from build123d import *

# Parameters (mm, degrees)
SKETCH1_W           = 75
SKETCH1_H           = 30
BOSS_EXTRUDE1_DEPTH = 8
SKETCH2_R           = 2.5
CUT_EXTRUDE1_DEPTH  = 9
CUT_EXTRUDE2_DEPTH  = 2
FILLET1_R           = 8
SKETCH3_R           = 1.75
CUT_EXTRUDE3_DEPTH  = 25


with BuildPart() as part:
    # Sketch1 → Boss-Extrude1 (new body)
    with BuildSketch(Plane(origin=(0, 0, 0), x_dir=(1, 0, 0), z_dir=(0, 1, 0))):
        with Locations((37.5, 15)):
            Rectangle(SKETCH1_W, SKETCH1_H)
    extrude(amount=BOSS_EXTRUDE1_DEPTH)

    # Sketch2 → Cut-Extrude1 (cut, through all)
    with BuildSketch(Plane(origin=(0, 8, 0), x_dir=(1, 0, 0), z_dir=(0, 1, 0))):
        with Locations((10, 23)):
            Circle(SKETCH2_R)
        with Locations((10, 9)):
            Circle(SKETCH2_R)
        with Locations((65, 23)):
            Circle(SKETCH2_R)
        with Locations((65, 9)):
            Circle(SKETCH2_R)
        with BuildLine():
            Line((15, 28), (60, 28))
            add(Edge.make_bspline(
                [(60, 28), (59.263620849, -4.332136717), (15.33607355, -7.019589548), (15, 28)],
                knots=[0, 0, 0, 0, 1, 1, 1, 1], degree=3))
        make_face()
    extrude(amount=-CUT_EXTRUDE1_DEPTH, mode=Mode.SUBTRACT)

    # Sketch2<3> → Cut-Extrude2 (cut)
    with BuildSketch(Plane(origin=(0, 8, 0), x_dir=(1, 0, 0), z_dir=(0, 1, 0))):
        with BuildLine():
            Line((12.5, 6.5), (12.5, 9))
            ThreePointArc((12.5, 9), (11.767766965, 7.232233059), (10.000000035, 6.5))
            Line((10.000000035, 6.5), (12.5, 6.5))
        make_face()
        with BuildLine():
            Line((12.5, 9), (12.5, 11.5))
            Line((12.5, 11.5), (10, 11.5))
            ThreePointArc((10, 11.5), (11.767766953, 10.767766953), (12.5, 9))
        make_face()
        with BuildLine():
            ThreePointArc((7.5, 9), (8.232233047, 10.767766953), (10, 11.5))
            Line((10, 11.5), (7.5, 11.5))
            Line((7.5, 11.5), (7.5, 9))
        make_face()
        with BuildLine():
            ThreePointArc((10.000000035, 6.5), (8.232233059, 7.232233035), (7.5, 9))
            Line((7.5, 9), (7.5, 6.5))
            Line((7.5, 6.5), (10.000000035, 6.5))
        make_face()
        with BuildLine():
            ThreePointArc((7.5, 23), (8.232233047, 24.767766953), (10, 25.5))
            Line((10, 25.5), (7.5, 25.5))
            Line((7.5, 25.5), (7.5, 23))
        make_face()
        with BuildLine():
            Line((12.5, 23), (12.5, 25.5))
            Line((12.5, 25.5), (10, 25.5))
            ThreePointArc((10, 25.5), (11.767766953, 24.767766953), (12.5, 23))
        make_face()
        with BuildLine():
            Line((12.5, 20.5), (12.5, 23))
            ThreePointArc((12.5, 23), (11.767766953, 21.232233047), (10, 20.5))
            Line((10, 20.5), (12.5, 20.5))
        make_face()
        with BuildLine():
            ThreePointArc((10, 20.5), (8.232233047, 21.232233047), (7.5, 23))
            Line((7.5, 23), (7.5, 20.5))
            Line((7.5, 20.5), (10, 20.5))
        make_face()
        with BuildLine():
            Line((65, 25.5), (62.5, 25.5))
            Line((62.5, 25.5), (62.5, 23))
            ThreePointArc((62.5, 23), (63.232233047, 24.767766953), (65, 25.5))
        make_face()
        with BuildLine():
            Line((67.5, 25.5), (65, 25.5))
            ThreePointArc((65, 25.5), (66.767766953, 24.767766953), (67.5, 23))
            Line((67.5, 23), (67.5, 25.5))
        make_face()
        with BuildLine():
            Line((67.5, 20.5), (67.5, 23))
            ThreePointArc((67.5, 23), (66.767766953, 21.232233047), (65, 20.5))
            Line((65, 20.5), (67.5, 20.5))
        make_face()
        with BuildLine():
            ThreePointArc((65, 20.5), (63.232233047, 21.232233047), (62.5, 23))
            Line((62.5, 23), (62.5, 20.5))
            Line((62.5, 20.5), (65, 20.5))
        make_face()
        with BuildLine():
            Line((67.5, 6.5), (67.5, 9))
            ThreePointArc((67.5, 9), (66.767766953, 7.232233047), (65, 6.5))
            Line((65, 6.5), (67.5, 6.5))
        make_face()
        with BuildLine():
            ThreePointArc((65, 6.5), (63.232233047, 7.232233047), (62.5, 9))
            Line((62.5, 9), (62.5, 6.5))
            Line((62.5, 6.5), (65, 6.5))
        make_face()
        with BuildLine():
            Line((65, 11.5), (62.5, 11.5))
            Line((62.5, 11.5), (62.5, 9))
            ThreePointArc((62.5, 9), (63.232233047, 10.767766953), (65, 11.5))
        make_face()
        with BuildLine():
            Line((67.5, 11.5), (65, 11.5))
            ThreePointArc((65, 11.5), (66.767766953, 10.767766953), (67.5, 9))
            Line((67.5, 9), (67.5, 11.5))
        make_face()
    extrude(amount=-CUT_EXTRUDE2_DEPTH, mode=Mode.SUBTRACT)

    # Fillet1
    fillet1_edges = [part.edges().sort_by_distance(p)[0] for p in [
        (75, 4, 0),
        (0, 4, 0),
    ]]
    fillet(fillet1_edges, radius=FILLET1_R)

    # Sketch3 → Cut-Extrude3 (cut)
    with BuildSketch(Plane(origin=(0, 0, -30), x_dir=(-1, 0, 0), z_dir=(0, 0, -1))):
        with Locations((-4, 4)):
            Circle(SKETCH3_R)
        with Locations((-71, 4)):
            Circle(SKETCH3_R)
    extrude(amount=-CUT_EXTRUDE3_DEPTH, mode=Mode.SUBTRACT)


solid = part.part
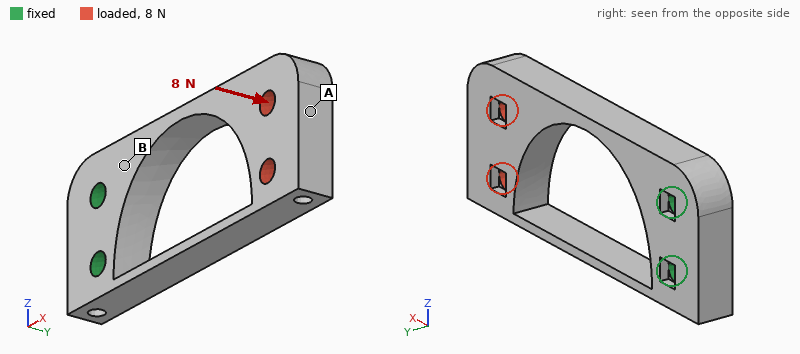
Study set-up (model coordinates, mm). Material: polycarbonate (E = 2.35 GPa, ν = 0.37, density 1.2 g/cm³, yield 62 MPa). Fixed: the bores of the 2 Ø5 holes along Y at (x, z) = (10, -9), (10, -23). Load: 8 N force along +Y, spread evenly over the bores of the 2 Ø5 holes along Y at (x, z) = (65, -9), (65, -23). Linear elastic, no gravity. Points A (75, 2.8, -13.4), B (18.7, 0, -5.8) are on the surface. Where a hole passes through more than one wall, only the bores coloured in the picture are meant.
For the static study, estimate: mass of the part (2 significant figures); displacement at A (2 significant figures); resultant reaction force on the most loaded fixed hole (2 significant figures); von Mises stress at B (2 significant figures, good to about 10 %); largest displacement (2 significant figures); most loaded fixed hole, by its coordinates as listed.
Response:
11 g
0.78 mm
5.6 N
2.3 MPa
0.87 mm
(10, -9)
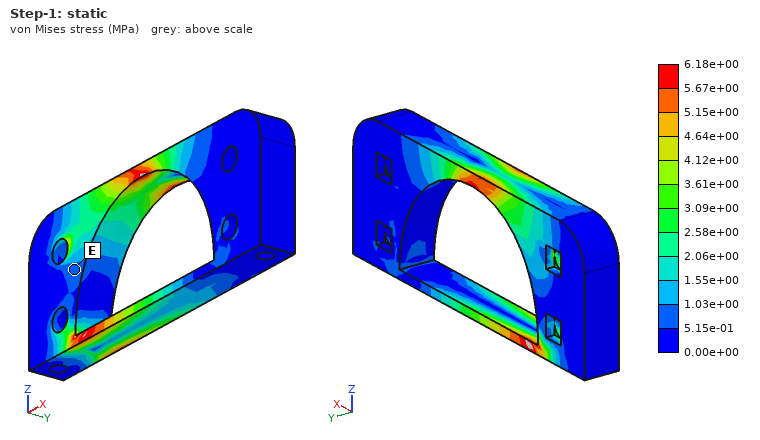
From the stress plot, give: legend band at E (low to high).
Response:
5.15e-01 to 1.03e+00 MPa
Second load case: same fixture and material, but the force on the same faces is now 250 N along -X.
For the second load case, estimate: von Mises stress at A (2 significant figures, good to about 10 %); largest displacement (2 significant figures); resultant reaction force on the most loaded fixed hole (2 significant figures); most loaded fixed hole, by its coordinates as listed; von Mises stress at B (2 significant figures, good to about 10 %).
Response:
2.8 MPa
0.76 mm
130 N
(10, -9)
3.3 MPa
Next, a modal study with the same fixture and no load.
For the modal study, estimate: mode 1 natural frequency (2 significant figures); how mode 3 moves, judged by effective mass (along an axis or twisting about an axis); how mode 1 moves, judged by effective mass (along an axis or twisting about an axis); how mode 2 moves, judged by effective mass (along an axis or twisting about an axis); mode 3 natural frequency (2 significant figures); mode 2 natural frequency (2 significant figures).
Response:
260 Hz
twisting about X
along Y
along Z
820 Hz
490 Hz
